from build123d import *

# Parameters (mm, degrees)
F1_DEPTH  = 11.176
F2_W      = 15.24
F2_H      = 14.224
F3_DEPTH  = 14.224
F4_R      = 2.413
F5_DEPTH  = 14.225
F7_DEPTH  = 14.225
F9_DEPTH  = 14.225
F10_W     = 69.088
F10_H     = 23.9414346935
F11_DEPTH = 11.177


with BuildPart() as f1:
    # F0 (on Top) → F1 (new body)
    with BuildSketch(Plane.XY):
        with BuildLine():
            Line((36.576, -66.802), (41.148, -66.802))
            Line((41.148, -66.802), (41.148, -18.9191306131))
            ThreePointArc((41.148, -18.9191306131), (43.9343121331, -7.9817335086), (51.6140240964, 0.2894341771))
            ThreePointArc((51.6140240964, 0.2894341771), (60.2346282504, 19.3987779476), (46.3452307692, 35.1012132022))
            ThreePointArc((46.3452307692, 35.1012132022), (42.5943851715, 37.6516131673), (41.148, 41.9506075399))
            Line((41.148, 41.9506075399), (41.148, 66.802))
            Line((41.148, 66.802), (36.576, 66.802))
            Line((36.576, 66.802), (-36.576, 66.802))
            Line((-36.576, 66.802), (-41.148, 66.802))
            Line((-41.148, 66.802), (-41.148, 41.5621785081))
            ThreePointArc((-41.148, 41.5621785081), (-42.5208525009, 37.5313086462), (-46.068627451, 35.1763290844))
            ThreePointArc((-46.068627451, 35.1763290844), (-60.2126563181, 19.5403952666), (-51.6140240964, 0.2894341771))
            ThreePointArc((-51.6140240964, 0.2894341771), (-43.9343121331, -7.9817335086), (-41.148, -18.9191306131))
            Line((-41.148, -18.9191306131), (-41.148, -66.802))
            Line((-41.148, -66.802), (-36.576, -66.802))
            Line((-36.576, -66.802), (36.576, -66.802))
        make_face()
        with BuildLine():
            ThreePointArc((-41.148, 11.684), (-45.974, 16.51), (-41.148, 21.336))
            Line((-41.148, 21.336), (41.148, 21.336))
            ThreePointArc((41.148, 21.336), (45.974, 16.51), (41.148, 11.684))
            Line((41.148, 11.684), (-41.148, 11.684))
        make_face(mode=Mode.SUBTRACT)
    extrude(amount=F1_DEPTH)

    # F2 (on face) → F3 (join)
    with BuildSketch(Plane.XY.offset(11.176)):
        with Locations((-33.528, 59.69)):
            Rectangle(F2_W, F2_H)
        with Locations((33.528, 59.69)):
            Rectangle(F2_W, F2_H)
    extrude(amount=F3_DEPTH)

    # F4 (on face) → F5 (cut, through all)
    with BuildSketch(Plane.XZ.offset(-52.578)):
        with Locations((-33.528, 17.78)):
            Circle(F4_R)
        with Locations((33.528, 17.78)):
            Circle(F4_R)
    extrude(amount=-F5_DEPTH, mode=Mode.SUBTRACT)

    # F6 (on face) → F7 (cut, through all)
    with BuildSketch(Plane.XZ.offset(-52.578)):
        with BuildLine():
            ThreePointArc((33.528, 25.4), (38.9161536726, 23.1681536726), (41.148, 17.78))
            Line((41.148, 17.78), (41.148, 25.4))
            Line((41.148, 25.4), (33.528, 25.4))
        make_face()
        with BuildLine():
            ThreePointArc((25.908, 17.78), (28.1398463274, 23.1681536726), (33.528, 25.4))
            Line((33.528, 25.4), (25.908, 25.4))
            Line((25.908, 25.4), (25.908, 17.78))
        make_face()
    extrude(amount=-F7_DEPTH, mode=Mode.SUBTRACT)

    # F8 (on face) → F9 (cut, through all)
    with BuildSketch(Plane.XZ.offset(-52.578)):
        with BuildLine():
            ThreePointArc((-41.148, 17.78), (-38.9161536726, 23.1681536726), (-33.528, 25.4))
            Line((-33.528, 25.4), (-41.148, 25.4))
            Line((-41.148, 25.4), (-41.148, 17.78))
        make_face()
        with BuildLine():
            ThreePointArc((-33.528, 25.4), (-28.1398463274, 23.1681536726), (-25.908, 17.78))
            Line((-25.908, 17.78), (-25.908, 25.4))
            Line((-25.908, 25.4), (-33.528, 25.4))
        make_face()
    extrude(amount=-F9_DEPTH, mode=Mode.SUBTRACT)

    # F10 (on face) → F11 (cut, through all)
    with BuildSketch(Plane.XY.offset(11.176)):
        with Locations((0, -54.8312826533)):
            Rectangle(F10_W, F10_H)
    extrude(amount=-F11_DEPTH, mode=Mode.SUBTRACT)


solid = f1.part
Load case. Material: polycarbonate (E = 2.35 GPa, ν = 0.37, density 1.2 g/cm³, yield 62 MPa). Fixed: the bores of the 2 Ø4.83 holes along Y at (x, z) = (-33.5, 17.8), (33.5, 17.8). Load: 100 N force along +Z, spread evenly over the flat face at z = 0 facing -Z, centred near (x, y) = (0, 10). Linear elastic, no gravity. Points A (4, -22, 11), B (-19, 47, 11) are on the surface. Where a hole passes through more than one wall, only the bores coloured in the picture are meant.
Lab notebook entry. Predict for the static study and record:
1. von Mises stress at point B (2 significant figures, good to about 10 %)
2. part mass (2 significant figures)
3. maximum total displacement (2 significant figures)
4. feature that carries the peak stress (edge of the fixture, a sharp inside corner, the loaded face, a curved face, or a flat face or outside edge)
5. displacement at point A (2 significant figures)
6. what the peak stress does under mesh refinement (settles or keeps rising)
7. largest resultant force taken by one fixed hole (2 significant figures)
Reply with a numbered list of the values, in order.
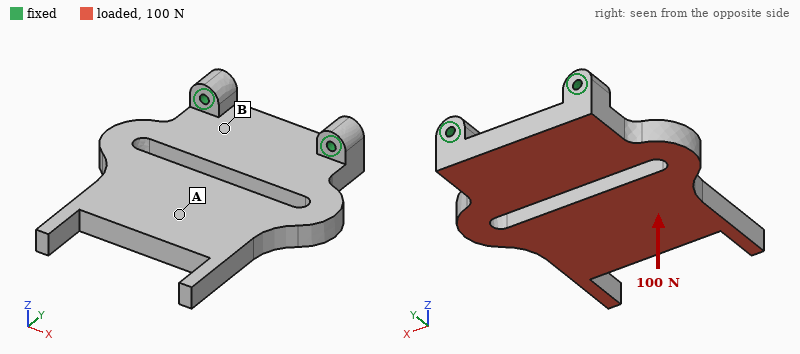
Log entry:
1. 1.6 MPa
2. 140 g
3. 2.2 mm
4. edge of the fixture
5. 1.2 mm
6. keeps rising
7. 53 N
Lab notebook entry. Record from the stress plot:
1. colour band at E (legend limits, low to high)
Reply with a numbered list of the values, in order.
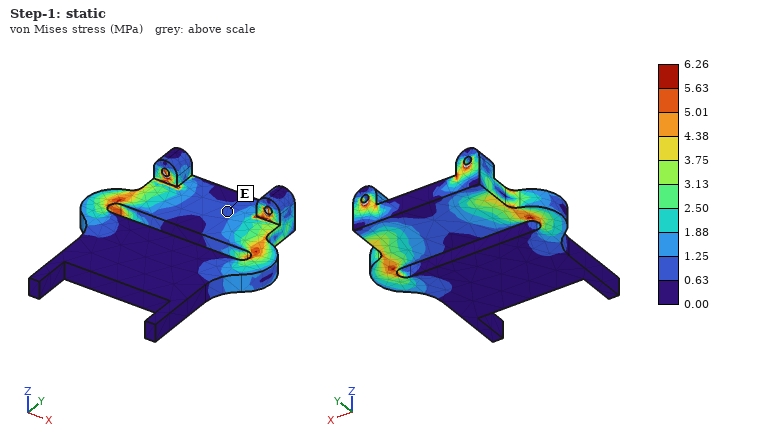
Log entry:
1. 0.63 to 1.25 MPa
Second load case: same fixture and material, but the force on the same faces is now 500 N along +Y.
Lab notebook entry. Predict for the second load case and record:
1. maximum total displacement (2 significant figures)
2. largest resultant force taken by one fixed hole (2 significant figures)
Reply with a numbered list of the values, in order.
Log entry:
1. 1.9 mm
2. 250 N
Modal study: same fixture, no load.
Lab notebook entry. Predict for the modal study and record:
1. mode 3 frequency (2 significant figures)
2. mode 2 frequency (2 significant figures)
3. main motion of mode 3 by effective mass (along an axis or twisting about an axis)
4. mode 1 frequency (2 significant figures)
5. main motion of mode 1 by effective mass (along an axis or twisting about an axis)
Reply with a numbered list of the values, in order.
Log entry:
1. 560 Hz
2. 460 Hz
3. along X
4. 130 Hz
5. along Z
